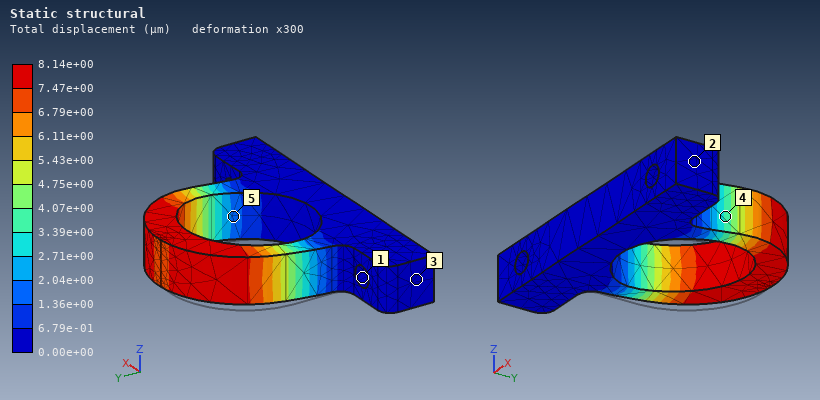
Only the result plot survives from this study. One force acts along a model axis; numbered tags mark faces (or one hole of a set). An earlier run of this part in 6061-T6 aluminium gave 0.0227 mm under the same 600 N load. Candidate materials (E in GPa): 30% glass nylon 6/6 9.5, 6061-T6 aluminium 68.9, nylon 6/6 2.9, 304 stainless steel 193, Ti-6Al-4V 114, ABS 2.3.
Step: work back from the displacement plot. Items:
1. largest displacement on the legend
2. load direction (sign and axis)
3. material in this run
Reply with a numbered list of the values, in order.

1. 8.14e+00 µm
2. +X
3. 304 stainless steel
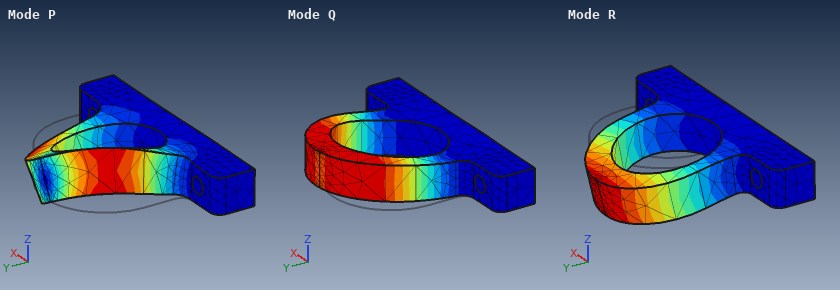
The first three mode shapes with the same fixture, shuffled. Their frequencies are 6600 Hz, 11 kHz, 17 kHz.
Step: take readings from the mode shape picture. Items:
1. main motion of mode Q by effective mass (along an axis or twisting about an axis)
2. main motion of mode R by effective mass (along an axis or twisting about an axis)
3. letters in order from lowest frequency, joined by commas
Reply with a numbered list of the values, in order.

1. along X
2. along Z
3. R, Q, P
